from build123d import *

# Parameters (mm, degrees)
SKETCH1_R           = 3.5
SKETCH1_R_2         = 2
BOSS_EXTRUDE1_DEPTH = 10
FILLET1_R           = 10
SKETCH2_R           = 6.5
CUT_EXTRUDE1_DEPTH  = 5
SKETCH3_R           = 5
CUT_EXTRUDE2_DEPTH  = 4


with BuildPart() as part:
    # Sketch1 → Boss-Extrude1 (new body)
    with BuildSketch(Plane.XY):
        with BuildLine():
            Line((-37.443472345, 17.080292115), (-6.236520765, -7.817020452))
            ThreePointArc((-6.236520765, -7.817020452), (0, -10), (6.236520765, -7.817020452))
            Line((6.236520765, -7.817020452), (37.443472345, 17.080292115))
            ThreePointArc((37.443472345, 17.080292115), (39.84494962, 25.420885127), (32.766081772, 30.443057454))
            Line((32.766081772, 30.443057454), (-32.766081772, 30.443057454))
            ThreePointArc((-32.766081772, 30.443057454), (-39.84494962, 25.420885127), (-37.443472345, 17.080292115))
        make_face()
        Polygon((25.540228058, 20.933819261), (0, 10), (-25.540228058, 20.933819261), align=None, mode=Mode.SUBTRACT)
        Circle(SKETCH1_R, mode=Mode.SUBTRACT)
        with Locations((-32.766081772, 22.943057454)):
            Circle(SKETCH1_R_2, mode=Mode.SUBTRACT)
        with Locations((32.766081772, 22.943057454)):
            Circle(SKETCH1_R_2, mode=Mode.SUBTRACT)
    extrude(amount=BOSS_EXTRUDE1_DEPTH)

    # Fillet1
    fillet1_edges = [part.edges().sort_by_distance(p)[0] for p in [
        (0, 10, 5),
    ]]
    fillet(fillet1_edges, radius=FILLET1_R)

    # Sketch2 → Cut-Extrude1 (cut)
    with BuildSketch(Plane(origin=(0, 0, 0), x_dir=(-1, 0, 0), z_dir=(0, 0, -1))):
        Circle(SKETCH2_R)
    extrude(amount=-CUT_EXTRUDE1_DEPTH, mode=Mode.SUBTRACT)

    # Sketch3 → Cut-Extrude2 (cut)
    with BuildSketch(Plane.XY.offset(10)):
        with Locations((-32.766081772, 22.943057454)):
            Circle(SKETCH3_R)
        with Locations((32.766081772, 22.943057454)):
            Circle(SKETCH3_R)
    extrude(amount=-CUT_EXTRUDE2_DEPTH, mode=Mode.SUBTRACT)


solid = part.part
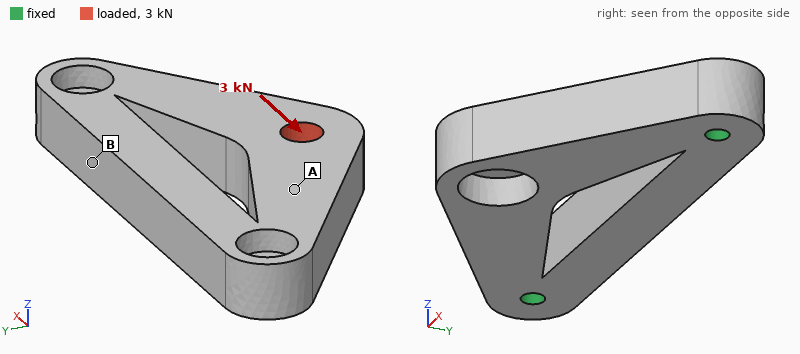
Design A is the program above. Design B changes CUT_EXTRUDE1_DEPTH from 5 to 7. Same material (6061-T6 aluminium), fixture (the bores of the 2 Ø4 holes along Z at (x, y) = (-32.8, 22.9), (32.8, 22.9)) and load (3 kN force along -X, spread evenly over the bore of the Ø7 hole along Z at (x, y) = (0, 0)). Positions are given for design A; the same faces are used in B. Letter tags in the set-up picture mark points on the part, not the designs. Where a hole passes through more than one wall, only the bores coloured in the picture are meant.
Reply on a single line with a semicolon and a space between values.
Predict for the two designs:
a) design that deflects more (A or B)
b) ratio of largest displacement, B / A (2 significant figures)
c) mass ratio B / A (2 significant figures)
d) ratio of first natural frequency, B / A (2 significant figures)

B; 1.2; 0.99; 1.0
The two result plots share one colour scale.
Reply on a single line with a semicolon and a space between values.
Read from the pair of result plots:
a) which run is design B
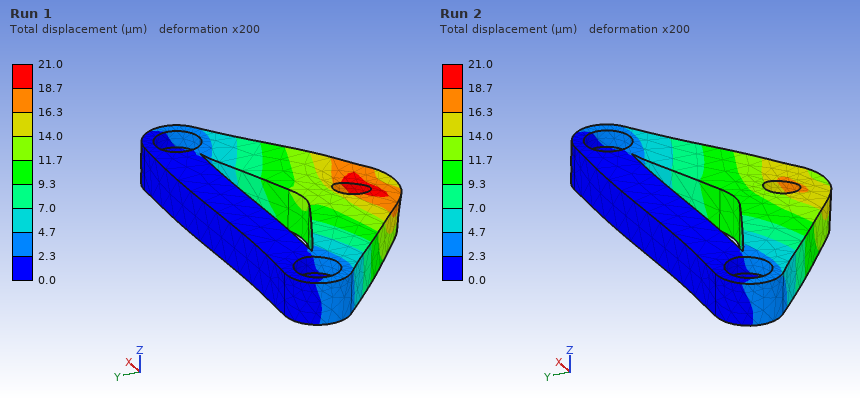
Run 1
